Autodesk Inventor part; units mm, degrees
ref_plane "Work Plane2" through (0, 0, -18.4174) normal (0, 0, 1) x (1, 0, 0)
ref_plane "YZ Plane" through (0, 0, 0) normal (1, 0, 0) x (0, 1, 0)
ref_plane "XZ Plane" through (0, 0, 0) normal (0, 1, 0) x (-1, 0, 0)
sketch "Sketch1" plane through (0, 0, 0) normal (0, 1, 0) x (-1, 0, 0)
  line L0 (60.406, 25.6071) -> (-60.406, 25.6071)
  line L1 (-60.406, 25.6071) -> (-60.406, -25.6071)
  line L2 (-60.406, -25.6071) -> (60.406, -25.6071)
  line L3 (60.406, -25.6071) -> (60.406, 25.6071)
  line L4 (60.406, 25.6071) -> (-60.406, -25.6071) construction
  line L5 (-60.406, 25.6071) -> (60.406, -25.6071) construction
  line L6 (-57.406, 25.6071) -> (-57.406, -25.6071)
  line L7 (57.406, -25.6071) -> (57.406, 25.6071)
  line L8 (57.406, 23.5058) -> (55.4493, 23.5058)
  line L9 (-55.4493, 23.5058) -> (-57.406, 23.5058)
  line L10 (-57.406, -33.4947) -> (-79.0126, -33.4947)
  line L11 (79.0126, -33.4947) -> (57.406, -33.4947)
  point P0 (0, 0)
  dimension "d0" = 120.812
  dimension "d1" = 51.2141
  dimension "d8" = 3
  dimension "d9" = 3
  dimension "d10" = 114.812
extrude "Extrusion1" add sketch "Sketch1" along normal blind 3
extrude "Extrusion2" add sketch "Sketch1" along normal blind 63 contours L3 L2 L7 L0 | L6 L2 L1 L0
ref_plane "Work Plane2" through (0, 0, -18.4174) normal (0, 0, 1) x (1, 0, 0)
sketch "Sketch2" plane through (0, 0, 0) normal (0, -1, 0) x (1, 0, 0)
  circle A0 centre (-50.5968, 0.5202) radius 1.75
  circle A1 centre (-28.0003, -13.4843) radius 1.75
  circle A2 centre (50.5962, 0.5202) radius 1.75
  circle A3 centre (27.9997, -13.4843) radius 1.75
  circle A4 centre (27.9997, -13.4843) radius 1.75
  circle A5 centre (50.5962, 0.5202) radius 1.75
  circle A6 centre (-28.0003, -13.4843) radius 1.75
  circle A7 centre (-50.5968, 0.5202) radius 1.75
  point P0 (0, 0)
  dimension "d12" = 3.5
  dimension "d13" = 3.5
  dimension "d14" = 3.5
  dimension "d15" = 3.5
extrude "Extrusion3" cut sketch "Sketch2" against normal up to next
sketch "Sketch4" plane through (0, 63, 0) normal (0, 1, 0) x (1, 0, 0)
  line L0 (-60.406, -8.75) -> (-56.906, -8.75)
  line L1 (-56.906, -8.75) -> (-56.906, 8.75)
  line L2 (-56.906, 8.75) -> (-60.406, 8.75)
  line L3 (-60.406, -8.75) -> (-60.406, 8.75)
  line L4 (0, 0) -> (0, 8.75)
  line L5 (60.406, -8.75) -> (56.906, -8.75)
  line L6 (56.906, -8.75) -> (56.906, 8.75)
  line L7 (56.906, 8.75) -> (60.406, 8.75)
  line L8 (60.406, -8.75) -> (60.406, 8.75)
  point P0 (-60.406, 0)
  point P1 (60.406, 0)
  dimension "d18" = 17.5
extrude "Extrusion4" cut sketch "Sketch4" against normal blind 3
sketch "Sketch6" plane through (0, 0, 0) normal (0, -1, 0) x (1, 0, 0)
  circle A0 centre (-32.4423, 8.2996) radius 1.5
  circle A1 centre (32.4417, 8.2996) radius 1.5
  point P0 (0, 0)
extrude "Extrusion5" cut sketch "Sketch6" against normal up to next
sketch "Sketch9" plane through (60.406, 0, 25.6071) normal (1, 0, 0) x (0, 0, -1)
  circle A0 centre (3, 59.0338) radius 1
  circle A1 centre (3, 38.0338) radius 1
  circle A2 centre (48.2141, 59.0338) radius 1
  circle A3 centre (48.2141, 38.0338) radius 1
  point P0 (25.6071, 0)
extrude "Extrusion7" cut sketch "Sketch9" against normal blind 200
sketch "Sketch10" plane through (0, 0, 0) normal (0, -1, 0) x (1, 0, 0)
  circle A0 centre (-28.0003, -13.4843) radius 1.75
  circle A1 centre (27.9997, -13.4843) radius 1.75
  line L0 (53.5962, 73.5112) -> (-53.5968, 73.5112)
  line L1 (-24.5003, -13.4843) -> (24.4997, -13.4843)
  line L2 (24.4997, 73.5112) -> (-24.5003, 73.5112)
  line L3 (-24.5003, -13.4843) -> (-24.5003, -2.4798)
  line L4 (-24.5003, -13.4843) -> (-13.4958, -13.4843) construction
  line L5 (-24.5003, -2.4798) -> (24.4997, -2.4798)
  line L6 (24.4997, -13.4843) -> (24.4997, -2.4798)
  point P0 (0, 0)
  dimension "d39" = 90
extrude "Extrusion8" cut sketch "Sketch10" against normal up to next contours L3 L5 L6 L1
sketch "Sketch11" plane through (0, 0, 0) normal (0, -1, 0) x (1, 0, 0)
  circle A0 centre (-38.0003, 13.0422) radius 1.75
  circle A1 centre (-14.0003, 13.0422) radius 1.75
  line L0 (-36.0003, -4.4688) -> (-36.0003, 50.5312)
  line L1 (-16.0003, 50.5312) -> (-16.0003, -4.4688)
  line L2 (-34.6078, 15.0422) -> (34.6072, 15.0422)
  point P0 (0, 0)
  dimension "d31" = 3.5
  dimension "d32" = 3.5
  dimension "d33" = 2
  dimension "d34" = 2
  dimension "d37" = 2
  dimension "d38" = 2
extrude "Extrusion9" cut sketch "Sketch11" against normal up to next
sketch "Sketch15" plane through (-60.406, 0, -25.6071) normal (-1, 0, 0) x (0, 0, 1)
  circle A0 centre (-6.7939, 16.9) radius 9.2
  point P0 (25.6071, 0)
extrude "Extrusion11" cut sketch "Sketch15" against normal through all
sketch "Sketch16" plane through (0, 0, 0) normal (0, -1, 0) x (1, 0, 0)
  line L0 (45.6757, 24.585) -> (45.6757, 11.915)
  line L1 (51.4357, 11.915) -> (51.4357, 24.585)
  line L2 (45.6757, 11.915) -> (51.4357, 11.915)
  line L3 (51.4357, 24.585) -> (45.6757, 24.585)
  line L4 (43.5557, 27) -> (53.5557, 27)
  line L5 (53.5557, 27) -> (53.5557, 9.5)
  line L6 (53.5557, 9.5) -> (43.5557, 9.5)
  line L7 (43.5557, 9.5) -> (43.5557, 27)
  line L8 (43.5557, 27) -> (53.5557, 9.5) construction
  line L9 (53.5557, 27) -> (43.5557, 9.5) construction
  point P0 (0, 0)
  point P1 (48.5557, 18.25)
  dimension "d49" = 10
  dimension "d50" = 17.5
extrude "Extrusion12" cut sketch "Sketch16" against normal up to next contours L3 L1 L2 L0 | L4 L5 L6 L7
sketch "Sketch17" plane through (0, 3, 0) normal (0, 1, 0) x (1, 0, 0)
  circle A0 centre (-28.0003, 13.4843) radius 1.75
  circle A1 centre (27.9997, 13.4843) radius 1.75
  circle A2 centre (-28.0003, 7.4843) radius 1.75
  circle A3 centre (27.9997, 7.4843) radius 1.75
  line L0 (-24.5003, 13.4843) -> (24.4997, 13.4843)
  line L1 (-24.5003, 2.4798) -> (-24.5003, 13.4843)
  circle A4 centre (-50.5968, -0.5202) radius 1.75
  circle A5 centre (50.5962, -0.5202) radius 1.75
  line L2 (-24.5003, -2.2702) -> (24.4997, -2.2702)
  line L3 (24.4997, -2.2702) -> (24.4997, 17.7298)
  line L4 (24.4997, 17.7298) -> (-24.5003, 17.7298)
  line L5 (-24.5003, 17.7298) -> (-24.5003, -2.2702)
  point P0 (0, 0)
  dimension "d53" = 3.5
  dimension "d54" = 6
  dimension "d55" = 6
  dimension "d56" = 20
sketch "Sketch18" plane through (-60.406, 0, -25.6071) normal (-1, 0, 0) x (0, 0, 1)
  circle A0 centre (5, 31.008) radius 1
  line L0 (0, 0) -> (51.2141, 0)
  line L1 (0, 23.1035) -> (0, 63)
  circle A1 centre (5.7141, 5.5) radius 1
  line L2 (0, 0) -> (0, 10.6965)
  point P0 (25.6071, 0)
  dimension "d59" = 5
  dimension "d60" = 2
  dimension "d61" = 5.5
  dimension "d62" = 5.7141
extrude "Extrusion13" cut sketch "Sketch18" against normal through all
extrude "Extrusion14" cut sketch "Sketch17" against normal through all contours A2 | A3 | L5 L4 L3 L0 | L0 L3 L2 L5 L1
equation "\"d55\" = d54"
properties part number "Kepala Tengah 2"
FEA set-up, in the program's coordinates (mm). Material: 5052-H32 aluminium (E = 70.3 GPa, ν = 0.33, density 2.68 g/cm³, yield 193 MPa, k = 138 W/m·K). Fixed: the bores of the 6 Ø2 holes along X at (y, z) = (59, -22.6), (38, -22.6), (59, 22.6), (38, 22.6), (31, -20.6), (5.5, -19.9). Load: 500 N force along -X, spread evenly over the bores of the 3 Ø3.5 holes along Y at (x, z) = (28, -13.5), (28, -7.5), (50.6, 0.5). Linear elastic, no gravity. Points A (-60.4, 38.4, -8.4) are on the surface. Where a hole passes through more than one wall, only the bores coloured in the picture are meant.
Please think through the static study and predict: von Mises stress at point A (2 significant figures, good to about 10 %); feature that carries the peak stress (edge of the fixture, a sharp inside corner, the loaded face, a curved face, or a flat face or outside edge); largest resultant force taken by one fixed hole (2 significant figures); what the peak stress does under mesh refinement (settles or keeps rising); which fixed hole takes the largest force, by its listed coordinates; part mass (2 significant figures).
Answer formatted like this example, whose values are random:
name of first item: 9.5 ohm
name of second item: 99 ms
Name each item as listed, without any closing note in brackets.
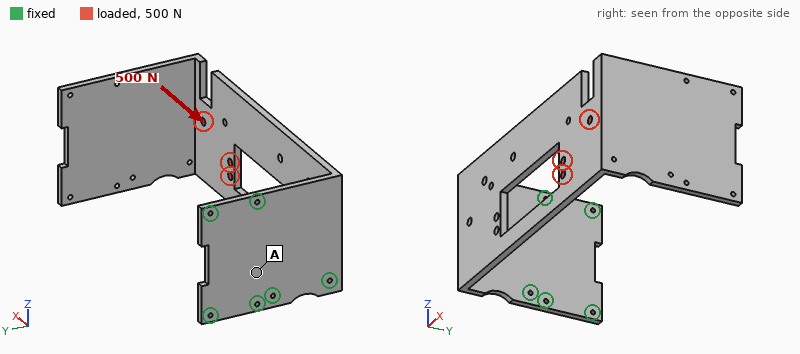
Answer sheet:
von Mises stress at point A: 7.9 MPa
feature that carries the peak stress: edge of the fixture
largest resultant force taken by one fixed hole: 480 N
what the peak stress does under mesh refinement: keeps rising
which fixed hole takes the largest force, by its listed coordinates: (5.5, -19.9)
part mass: 88 g
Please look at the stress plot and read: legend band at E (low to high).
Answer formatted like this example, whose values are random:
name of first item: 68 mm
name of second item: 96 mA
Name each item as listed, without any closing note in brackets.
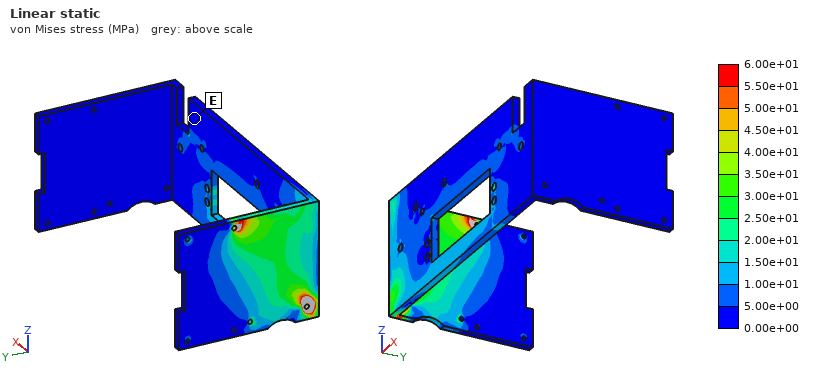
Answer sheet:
legend band at E: 0.00e+00 to 5.00e+00 MPa
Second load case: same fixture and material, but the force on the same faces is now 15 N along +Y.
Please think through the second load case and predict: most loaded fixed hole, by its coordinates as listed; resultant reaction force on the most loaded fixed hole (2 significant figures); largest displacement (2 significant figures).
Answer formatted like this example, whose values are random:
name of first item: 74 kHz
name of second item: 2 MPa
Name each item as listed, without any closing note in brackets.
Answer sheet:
most loaded fixed hole, by its coordinates as listed: (5.5, -19.9)
resultant reaction force on the most loaded fixed hole: 33 N
largest displacement: 1.4 mm
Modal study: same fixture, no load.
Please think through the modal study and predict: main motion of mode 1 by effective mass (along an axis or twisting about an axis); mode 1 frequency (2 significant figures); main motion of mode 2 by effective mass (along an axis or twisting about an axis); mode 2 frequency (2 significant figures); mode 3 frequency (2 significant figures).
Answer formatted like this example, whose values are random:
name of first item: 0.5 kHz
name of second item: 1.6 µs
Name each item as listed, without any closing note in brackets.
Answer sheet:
main motion of mode 1 by effective mass: along Y
mode 1 frequency: 79 Hz
main motion of mode 2 by effective mass: along Z
mode 2 frequency: 180 Hz
mode 3 frequency: 320 Hz
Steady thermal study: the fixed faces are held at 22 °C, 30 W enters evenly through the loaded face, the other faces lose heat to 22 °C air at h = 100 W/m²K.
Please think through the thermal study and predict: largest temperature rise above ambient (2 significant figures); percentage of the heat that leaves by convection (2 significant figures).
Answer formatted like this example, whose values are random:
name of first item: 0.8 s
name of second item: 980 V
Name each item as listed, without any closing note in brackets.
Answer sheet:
largest temperature rise above ambient: 56 K
percentage of the heat that leaves by convection: 94 %
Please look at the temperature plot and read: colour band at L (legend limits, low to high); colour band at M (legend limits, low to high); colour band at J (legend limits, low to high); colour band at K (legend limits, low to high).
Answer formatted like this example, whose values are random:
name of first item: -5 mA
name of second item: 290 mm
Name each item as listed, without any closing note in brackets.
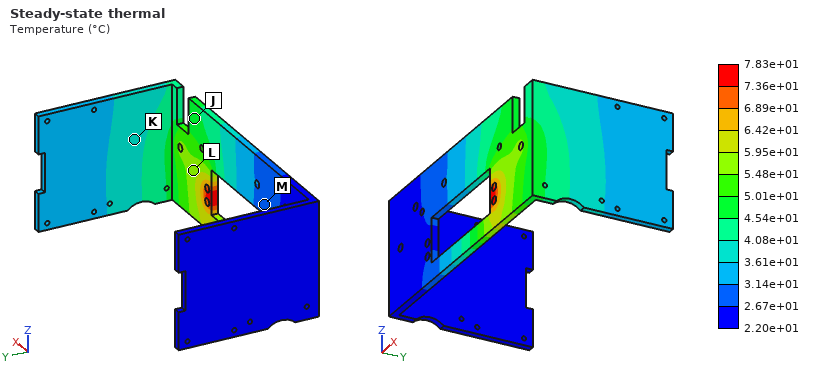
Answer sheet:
colour band at L: 5.48e+01 to 5.95e+01 °C
colour band at M: 2.67e+01 to 3.14e+01 °C
colour band at J: 4.54e+01 to 5.01e+01 °C
colour band at K: 3.61e+01 to 4.08e+01 °C
